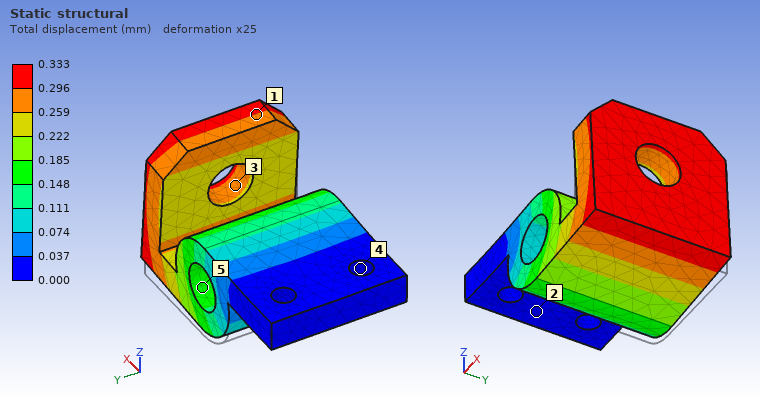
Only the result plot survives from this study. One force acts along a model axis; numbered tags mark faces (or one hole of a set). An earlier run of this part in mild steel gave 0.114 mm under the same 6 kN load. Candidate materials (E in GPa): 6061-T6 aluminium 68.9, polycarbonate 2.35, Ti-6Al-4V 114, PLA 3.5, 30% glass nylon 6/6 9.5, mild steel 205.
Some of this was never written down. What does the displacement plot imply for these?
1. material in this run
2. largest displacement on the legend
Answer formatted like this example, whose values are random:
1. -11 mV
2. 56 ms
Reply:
1. 6061-T6 aluminium
2. 0.333 mm
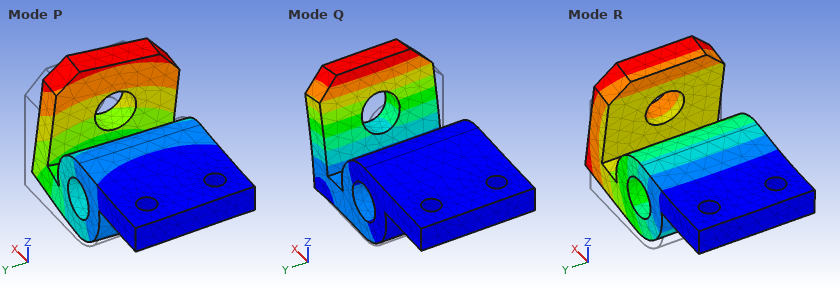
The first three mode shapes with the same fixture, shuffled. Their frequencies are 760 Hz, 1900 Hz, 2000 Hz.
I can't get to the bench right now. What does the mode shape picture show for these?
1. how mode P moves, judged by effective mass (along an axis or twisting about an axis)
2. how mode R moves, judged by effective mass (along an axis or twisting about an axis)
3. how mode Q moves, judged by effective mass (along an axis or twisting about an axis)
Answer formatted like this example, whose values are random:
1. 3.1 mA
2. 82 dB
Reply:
1. along Y
2. along Z
3. along X
